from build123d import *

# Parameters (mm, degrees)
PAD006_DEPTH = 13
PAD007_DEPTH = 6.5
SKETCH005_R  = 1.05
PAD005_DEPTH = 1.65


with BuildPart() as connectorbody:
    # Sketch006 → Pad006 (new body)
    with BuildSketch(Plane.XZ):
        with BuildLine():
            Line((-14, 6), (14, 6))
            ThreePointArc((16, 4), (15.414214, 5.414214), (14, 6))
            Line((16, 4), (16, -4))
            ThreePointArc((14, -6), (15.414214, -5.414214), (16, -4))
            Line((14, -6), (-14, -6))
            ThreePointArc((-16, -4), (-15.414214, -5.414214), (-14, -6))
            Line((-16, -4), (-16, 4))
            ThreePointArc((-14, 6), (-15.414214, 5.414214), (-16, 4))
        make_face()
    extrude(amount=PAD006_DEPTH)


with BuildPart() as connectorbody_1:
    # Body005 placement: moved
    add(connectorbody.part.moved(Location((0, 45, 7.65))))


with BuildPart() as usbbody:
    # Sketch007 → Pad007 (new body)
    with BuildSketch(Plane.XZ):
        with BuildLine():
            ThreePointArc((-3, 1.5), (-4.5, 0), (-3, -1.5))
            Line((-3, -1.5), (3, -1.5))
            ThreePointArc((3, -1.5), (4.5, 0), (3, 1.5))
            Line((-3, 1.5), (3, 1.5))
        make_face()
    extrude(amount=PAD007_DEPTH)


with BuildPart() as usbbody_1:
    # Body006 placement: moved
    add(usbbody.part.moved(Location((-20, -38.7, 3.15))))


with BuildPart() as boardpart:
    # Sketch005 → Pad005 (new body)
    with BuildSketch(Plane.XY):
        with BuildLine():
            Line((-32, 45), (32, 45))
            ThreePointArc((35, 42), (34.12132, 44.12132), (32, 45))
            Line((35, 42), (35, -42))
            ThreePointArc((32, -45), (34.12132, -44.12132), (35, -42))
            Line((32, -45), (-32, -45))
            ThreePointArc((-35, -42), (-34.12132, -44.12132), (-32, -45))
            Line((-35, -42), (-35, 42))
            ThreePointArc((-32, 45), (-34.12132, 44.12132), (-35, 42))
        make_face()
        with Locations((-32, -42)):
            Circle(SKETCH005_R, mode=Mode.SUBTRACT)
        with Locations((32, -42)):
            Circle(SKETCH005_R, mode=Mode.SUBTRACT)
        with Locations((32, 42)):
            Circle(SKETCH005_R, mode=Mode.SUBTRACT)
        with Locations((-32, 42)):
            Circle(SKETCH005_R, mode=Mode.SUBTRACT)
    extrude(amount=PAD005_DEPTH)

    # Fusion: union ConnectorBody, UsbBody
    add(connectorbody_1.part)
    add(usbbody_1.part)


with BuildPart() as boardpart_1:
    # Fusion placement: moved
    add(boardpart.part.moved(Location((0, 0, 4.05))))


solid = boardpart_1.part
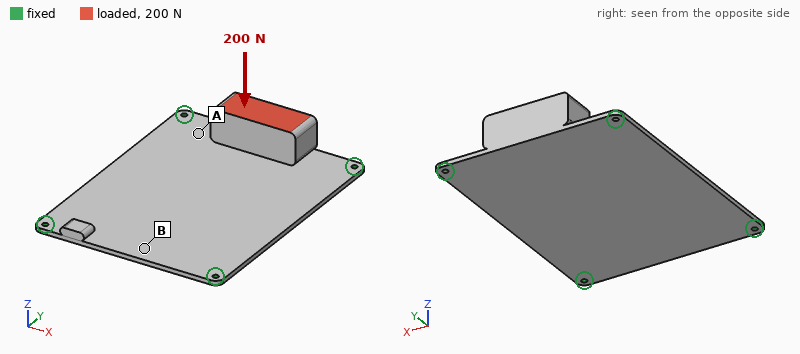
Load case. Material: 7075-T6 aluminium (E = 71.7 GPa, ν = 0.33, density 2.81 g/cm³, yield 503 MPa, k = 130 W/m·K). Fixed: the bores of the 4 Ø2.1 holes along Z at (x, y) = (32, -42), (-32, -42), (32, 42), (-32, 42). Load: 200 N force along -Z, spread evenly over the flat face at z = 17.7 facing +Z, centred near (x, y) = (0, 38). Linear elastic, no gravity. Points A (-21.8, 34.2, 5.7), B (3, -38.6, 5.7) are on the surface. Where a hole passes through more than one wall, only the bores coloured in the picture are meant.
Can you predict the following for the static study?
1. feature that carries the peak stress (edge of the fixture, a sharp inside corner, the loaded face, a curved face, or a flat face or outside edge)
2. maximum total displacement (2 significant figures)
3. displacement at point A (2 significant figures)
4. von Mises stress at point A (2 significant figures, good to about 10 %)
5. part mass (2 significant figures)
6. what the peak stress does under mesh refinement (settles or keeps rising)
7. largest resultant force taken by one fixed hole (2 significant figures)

edge of the fixture
0.15 mm
0.087 mm
36 MPa
43 g
keeps rising
110 N
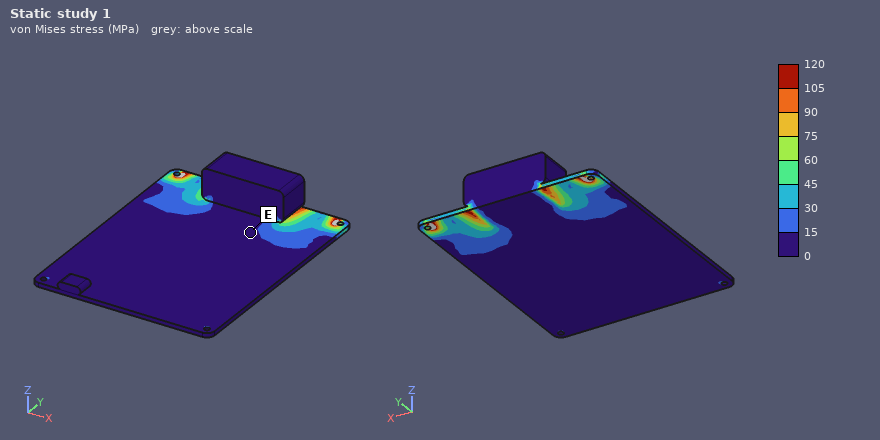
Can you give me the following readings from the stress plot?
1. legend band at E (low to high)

0 to 15 MPa
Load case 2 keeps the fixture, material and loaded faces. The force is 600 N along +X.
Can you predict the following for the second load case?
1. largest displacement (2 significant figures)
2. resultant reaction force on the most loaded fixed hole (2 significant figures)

0.17 mm
300 N
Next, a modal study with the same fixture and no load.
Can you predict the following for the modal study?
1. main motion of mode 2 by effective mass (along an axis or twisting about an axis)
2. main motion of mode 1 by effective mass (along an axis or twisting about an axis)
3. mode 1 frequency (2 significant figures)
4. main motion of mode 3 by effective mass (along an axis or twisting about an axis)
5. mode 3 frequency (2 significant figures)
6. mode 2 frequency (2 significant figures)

along Z
along Z
840 Hz
twisting about Y
1600 Hz
1400 Hz
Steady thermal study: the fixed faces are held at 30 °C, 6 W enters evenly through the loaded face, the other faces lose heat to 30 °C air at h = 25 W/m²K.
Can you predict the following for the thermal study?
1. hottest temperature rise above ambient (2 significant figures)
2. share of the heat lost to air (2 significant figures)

13 K
30 %
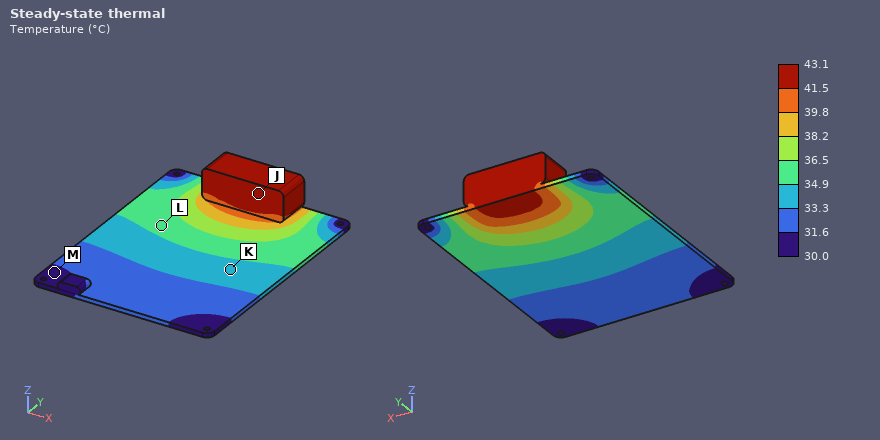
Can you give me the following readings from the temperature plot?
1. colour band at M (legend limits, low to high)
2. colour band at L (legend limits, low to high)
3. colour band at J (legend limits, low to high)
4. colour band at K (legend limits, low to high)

30.0 to 31.6 °C
34.9 to 36.5 °C
41.5 to 43.1 °C
33.3 to 34.9 °C
